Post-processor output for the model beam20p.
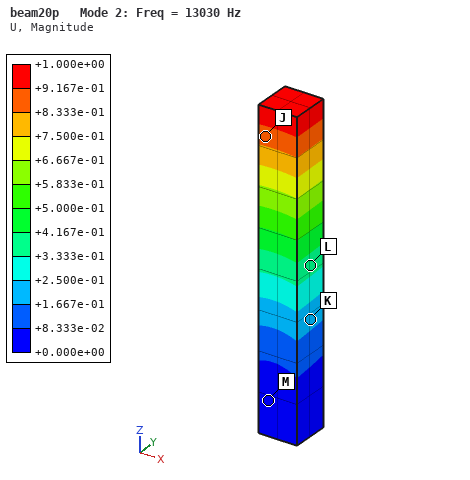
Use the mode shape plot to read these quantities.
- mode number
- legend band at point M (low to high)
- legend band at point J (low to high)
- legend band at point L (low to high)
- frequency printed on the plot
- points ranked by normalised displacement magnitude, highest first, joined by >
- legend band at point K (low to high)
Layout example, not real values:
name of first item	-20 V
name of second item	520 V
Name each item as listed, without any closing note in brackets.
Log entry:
mode number	2
legend band at point M	+0.000e+00 to +8.333e-02
legend band at point J	+8.333e-01 to +9.167e-01
legend band at point L	+3.333e-01 to +4.167e-01
frequency printed on the plot	13030 Hz
points ranked by normalised displacement magnitude, highest first, joined by >	J > L > K > M
legend band at point K	+1.667e-01 to +2.500e-01
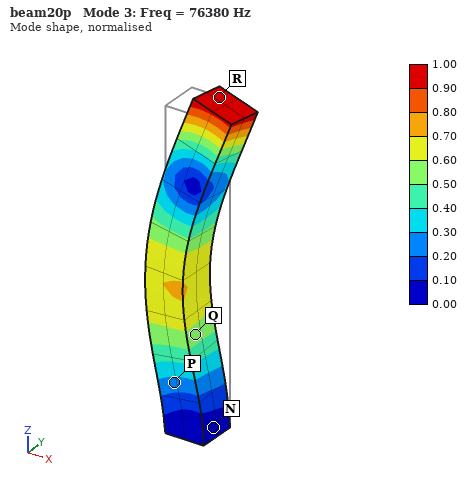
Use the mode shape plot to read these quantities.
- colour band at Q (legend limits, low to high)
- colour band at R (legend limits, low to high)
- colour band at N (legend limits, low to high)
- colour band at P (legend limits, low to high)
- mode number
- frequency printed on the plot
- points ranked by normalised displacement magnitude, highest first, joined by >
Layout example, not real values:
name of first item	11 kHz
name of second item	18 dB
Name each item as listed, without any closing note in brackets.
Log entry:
colour band at Q	0.50 to 0.60
colour band at R	0.90 to 1.00
colour band at N	0.00 to 0.10
colour band at P	0.20 to 0.30
mode number	3
frequency printed on the plot	76380 Hz
points ranked by normalised displacement magnitude, highest first, joined by >	R > Q > P > N
